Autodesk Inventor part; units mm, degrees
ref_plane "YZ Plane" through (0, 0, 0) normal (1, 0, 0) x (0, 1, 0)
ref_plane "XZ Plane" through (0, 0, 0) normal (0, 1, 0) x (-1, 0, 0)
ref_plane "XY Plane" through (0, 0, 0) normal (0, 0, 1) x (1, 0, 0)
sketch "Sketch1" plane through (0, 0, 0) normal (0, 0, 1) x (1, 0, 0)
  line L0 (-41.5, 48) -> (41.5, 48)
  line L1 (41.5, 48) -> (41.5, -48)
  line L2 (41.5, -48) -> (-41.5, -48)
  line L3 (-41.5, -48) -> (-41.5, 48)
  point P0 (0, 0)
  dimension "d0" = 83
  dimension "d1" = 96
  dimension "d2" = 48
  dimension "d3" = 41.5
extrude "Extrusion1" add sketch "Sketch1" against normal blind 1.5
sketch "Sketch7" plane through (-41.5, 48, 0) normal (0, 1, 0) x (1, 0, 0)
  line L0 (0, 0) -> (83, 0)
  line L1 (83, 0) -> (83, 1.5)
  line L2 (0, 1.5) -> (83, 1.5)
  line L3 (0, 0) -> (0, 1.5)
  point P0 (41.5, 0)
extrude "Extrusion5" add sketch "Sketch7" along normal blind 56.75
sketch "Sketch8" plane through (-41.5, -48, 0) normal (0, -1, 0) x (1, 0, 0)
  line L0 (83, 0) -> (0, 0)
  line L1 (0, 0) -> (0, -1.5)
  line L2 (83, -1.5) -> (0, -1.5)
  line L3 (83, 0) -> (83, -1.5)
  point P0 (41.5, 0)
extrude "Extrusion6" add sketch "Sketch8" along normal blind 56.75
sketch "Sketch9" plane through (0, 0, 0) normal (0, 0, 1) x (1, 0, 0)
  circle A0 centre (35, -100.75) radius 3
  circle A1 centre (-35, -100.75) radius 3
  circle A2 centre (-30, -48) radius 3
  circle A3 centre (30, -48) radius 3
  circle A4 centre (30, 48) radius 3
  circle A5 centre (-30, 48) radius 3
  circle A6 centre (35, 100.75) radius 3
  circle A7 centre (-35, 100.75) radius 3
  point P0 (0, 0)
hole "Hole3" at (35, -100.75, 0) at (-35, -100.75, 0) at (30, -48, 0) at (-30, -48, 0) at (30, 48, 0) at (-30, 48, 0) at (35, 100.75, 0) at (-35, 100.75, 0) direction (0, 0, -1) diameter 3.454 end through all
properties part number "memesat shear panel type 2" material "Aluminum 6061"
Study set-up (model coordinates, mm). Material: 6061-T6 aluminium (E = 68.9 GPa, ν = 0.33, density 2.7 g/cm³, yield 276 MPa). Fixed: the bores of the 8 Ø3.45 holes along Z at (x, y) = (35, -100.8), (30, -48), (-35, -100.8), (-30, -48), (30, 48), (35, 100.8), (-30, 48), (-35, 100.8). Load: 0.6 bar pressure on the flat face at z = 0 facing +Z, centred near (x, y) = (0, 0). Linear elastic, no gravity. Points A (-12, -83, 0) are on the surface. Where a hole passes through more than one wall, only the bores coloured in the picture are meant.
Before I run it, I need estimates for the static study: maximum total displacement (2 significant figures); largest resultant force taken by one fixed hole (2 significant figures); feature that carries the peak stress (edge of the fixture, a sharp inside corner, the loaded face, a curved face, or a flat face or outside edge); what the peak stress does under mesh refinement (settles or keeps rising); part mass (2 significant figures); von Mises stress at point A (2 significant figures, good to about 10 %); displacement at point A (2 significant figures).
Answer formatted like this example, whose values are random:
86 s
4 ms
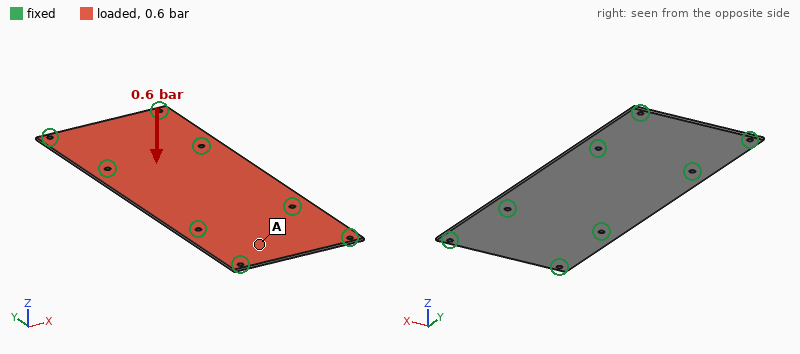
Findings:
0.83 mm
200 N
edge of the fixture
keeps rising
70 g
21 MPa
0.18 mm
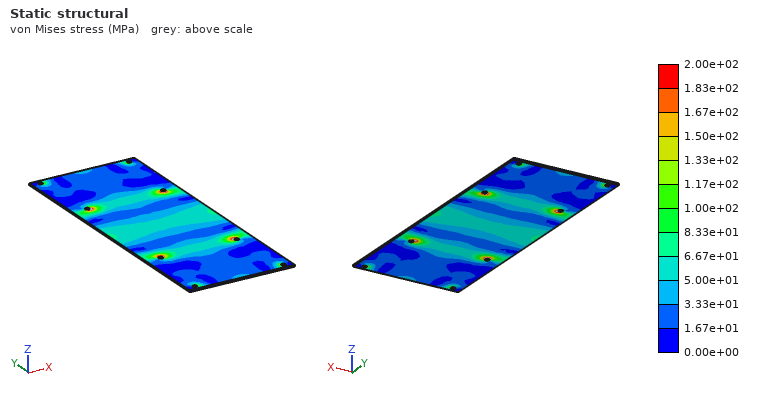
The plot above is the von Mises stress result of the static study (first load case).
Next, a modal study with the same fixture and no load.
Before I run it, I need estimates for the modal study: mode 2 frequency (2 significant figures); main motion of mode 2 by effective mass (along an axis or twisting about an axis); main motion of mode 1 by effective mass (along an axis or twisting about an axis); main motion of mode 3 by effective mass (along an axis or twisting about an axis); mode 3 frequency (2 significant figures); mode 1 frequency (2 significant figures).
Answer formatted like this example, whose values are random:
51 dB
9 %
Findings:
1100 Hz
twisting about Y
along Z
along Z
1500 Hz
770 Hz
